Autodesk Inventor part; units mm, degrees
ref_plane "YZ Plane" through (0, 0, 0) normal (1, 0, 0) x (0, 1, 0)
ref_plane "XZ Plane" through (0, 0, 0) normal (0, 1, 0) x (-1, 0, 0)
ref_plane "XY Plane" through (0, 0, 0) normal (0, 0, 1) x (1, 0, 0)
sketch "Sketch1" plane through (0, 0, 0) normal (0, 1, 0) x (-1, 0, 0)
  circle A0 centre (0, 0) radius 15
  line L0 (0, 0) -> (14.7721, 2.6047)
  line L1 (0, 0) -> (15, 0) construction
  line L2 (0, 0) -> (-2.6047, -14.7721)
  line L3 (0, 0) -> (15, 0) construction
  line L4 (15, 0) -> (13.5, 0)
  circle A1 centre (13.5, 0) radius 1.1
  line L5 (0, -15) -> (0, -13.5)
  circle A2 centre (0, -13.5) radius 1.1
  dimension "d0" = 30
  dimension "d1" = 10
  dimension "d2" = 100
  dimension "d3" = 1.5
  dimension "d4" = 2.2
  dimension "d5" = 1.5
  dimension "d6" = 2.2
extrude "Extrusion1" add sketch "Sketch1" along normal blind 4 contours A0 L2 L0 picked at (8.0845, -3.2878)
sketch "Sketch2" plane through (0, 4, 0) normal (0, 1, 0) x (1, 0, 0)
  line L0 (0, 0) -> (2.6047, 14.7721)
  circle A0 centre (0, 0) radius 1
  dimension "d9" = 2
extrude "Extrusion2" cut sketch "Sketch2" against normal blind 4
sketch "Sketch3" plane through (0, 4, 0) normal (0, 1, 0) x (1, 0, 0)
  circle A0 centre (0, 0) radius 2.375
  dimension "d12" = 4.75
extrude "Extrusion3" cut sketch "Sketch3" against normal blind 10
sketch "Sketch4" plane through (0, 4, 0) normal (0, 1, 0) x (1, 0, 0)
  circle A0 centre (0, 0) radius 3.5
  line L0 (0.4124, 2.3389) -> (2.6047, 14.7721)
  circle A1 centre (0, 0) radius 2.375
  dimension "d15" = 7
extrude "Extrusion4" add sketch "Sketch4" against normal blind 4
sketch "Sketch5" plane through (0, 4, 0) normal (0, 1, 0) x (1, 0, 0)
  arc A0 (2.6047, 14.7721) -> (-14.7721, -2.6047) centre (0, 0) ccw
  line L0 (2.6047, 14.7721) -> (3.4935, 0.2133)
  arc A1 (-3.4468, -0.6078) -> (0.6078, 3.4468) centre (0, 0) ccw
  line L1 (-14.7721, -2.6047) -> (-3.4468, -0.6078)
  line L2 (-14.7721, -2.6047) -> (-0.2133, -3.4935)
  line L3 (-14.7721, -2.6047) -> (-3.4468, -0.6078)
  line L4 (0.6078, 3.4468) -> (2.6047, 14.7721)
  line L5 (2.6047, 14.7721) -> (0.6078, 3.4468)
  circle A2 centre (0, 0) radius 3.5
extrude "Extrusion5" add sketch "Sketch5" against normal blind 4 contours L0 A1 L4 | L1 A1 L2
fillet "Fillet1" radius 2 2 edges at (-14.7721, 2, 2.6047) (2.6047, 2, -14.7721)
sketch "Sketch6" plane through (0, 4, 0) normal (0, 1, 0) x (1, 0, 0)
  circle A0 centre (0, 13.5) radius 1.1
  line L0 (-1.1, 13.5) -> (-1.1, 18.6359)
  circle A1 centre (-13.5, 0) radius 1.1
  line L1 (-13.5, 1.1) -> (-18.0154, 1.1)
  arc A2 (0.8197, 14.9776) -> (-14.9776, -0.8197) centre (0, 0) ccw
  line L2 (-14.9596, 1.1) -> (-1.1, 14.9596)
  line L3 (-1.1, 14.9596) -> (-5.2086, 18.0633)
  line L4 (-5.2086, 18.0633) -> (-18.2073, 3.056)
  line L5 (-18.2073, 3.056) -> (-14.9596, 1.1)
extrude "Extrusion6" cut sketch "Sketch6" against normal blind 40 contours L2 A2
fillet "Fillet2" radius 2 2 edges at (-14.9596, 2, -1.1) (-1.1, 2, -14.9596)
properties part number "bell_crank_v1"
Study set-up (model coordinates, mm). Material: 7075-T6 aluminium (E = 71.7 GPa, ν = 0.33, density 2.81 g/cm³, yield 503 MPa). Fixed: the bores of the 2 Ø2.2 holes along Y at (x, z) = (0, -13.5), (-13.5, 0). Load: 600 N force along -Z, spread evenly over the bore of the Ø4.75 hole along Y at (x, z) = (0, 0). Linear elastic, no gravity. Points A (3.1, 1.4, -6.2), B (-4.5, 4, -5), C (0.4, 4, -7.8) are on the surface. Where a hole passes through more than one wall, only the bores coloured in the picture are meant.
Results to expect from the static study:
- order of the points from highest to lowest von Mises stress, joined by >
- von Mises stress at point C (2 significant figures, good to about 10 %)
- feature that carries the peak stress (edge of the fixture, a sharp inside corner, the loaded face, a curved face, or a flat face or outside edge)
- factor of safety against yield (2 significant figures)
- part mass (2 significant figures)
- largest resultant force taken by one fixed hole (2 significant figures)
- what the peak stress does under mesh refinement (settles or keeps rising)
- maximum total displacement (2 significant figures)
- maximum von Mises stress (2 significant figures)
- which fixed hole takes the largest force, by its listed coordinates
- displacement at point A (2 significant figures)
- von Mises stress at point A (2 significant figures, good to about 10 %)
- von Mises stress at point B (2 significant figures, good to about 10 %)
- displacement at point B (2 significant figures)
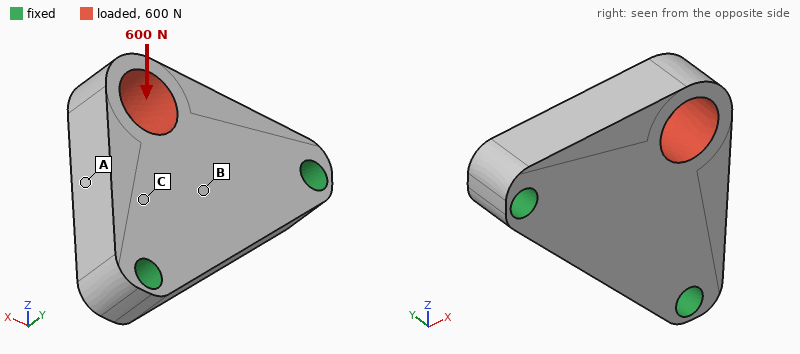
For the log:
A > C > B
22 MPa
the loaded face
5.7
2.3 g
540 N
settles
9.4 µm
88 MPa
(0, -13.5)
2.7 µm
36 MPa
9.4 MPa
2.4 µm
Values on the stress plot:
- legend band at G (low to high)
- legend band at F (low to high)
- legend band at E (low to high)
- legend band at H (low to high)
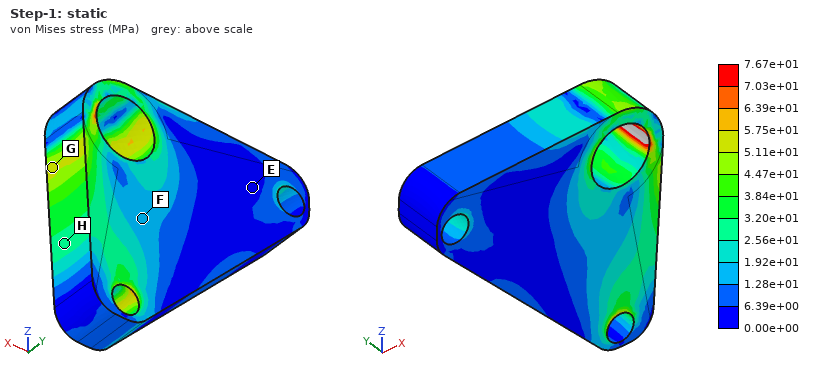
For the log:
5.11e+01 to 5.75e+01 MPa
1.28e+01 to 1.92e+01 MPa
0.00e+00 to 6.39e+00 MPa
2.56e+01 to 3.20e+01 MPa
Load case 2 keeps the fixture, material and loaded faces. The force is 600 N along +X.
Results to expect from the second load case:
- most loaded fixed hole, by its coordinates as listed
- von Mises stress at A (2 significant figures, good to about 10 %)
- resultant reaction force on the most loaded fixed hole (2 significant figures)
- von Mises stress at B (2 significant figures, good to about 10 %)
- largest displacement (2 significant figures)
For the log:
(-13.5, 0)
13 MPa
540 N
7.7 MPa
9.4 µm
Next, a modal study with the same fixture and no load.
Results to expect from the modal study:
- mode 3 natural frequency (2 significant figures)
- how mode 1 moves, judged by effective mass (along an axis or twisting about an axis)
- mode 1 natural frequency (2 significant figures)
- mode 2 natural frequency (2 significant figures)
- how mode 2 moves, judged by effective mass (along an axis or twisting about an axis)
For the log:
54 kHz
along Y
21 kHz
51 kHz
along Y
